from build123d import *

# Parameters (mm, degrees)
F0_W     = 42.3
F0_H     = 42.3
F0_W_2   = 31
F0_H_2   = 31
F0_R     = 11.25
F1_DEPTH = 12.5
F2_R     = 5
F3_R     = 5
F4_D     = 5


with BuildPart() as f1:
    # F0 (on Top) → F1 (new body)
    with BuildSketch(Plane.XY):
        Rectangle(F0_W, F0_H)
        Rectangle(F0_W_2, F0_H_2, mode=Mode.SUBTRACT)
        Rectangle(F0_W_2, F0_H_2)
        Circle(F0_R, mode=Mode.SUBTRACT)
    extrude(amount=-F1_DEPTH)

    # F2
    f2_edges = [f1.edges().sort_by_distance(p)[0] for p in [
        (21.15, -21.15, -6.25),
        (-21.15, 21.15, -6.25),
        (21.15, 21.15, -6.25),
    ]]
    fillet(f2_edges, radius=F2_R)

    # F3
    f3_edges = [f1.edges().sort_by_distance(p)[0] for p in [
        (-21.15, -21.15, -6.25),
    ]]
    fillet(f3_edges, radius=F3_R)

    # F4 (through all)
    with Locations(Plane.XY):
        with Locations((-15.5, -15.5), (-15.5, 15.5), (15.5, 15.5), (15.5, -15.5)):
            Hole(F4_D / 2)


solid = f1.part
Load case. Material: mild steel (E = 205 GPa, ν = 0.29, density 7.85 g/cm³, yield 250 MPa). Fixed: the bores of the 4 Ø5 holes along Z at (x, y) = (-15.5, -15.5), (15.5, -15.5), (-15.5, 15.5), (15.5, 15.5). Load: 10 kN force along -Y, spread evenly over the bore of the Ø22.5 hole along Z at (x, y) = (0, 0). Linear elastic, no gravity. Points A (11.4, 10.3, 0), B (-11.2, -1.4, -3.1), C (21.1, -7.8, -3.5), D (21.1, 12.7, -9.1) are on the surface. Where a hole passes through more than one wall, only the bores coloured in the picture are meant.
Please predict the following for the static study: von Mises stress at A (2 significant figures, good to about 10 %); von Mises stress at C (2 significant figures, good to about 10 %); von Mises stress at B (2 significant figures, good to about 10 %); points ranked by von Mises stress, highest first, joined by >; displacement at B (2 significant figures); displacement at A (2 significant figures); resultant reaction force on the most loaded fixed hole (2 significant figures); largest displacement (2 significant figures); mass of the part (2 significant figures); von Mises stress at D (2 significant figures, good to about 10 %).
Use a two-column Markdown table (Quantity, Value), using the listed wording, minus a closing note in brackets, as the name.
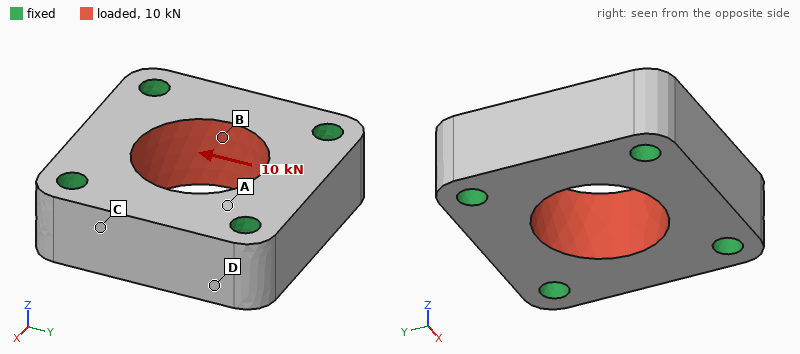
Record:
| Quantity | Value |
|---|---|
| von Mises stress at A | 17 MPa |
| von Mises stress at C | 8.0 MPa |
| von Mises stress at B | 20 MPa |
| points ranked by von Mises stress, highest first, joined by > | B > A > C > D |
| displacement at B | 0.90 µm |
| displacement at A | 0.66 µm |
| resultant reaction force on the most loaded fixed hole | 2.6 kN |
| largest displacement | 2.2 µm |
| mass of the part | 130 g |
| von Mises stress at D | 4.5 MPa |
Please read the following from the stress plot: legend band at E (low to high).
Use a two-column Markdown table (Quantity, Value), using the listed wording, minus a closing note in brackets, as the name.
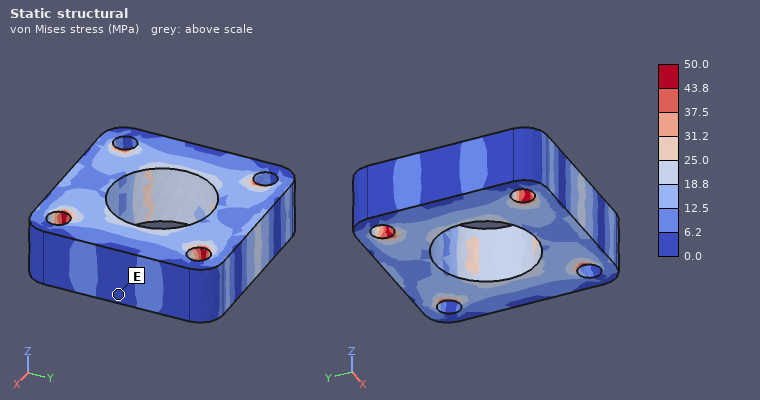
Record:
| Quantity | Value |
|---|---|
| legend band at E | 0.0 to 6.2 MPa |
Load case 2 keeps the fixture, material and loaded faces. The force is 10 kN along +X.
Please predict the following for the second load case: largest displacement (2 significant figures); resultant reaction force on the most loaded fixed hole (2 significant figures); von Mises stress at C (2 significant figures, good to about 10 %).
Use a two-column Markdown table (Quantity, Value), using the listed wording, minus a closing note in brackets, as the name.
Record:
| Quantity | Value |
|---|---|
| largest displacement | 2.2 µm |
| resultant reaction force on the most loaded fixed hole | 2.6 kN |
| von Mises stress at C | 5.1 MPa |
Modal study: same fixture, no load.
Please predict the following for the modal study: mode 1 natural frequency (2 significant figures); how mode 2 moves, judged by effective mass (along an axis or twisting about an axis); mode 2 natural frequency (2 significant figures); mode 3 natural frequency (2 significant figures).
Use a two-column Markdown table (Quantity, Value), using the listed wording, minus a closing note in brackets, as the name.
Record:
| Quantity | Value |
|---|---|
| mode 1 natural frequency | 34 kHz |
| how mode 2 moves, judged by effective mass | along Z |
| mode 2 natural frequency | 42 kHz |
| mode 3 natural frequency | 45 kHz |
